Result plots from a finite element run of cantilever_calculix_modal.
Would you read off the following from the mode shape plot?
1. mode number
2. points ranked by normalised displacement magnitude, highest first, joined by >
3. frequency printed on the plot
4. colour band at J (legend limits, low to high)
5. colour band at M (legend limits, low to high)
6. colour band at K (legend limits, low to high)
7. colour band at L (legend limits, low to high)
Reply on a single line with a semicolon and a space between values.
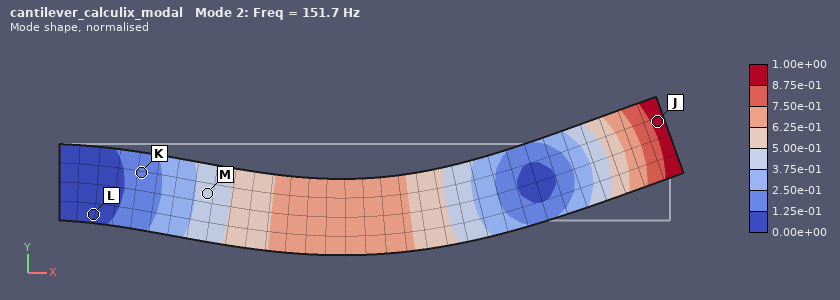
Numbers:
2; J > M > K > L; 151.7 Hz; 8.75e-01 to 1.00e+00; 3.75e-01 to 5.00e-01; 1.25e-01 to 2.50e-01; 0.00e+00 to 1.25e-01
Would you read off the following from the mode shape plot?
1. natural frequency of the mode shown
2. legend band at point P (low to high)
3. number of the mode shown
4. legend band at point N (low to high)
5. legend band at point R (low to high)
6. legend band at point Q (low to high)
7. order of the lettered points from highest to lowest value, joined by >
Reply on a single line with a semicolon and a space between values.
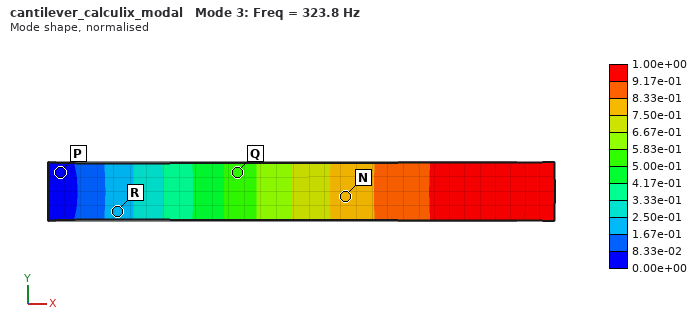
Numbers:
323.8 Hz; 0.00e+00 to 8.33e-02; 3; 7.50e-01 to 8.33e-01; 1.67e-01 to 2.50e-01; 5.00e-01 to 5.83e-01; N > Q > R > P
